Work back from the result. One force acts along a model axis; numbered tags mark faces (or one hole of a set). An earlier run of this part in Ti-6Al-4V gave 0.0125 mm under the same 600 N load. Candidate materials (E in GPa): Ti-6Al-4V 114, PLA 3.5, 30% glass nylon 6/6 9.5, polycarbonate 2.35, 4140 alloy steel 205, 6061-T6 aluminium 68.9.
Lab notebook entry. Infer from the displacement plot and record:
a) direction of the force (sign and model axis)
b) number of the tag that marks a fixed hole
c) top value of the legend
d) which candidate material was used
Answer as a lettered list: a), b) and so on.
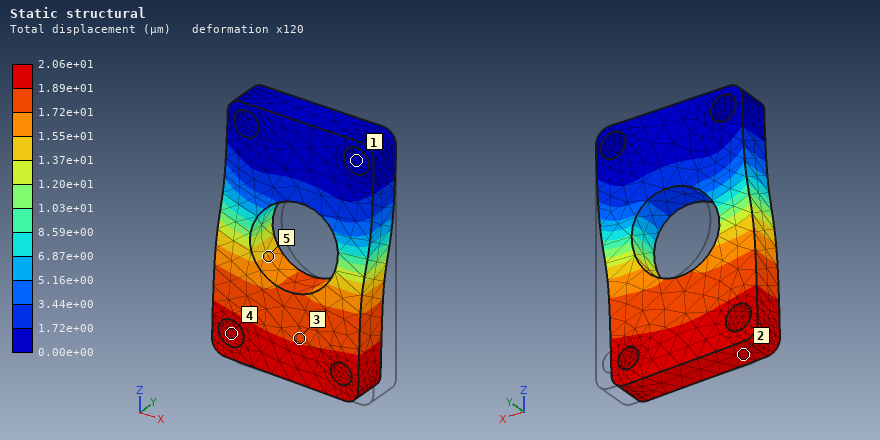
a) -X
b) 1
c) 2.06e+01 µm
d) 6061-T6 aluminium
